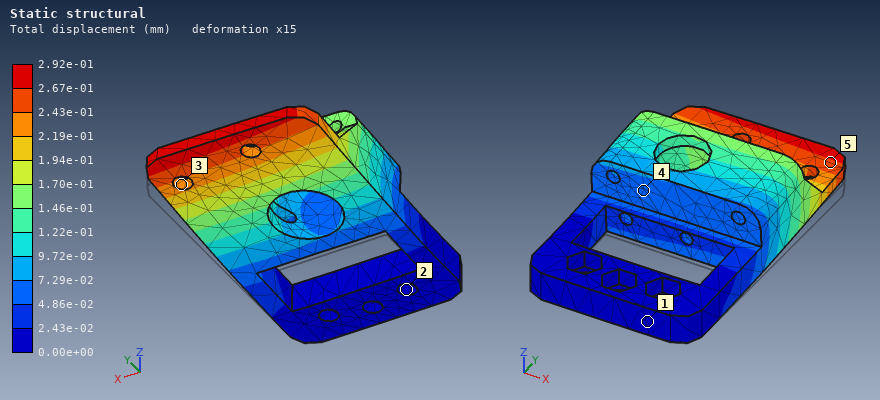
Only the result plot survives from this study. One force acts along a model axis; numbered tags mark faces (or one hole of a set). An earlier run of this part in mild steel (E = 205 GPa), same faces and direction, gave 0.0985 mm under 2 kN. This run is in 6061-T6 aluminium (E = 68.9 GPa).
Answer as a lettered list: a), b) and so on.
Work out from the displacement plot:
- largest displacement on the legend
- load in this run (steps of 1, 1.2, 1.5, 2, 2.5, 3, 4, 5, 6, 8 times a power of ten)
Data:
a) 2.92e-01 mm
b) 2 kN
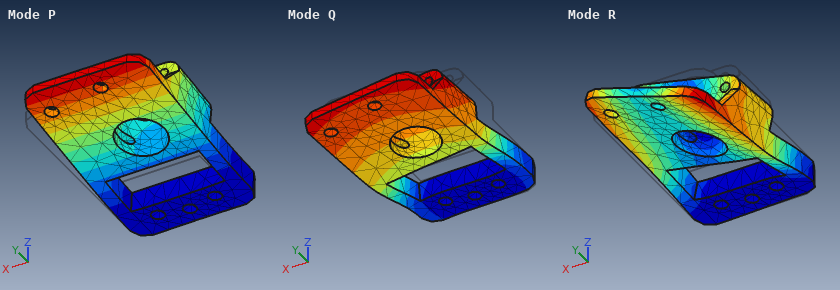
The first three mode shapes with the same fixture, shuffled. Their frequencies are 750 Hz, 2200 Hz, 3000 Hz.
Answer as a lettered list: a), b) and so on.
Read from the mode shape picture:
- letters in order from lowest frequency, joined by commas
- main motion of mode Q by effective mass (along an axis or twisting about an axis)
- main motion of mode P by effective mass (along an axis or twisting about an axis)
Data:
a) P, Q, R
b) along X
c) along Z
